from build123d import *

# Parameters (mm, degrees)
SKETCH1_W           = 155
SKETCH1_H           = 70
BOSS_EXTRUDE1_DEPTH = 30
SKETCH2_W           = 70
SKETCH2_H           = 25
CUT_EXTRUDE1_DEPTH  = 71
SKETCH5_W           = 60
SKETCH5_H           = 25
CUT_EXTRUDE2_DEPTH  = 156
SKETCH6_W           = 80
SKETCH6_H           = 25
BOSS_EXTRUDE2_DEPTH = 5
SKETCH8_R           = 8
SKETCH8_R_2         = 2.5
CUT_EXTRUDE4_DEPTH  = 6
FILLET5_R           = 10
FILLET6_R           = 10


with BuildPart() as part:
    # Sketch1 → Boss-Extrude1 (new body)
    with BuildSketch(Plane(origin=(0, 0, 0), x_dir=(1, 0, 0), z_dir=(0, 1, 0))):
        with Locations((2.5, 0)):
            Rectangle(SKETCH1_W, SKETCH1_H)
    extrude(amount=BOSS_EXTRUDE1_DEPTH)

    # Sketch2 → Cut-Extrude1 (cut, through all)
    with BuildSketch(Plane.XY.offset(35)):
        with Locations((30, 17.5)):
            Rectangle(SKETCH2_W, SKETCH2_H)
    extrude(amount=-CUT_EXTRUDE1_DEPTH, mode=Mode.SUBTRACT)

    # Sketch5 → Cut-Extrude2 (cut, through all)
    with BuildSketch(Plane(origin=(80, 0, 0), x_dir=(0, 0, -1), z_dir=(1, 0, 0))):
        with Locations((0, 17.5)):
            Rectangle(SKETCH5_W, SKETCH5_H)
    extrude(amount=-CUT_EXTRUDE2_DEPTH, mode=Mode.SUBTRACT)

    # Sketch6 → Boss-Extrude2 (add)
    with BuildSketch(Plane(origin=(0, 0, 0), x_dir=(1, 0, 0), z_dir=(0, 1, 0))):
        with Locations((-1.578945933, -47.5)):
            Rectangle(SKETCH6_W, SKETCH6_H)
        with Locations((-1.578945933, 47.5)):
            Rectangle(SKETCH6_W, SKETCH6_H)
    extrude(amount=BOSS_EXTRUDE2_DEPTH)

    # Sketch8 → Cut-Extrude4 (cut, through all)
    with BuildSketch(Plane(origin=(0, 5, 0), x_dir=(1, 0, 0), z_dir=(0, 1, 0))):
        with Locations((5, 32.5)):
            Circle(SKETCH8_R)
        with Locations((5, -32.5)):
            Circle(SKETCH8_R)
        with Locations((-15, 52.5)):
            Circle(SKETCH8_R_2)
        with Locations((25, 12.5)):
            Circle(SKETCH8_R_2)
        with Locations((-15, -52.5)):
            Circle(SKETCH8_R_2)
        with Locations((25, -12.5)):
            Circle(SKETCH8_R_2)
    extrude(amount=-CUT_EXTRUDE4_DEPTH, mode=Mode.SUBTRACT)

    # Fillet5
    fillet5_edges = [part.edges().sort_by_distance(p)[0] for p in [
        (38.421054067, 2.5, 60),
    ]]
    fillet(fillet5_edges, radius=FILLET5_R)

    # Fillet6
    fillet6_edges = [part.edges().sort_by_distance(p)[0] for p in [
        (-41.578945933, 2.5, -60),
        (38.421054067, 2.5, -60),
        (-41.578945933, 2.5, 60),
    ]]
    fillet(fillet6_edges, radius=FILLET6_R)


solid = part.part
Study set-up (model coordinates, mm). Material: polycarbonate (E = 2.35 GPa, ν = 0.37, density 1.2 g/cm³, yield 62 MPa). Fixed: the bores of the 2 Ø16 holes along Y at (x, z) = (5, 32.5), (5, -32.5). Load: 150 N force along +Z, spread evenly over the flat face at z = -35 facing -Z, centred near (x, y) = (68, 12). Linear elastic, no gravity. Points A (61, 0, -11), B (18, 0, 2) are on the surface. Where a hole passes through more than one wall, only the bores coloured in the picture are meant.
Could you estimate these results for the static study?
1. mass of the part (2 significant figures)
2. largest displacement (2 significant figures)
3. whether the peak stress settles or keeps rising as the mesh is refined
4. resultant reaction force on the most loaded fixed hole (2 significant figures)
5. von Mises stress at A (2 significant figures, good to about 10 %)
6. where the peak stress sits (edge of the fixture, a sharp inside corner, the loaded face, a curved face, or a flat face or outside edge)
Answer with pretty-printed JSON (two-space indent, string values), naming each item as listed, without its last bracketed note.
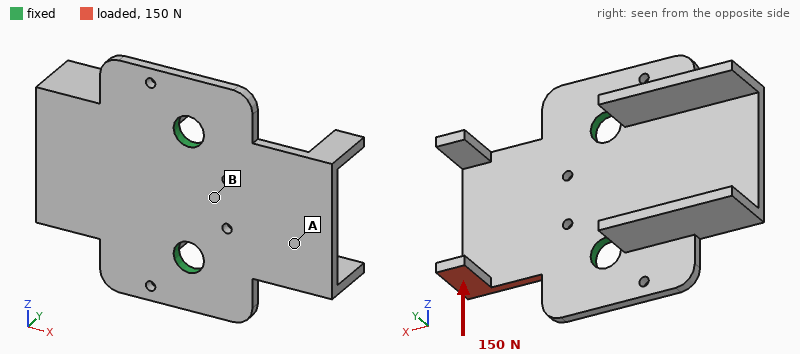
{
  "mass of the part": "110 g",
  "largest displacement": "2.4 mm",
  "whether the peak stress settles or keeps rising as the mesh is refined": "keeps rising",
  "resultant reaction force on the most loaded fixed hole": "150 N",
  "von Mises stress at A": "4.2 MPa",
  "where the peak stress sits": "a sharp inside corner"
}
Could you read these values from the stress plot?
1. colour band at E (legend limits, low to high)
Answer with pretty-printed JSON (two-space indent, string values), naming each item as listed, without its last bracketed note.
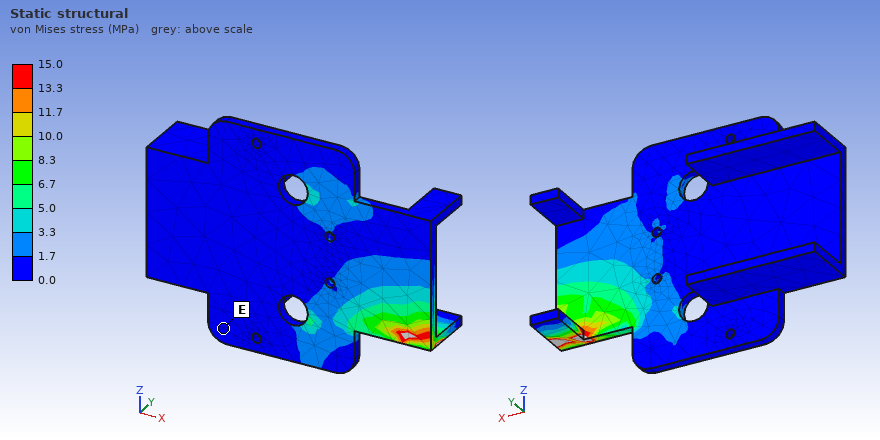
{
  "colour band at E": "0.0 to 1.7 MPa"
}
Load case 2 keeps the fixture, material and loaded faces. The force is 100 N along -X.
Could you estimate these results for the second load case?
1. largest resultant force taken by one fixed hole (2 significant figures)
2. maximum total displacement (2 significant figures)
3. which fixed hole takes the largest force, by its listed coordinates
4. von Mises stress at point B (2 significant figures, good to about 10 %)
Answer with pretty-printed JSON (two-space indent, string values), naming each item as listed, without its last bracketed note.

{
  "largest resultant force taken by one fixed hole": "100 N",
  "maximum total displacement": "2.1 mm",
  "which fixed hole takes the largest force, by its listed coordinates": "(5, -32.5)",
  "von Mises stress at point B": "1.9 MPa"
}
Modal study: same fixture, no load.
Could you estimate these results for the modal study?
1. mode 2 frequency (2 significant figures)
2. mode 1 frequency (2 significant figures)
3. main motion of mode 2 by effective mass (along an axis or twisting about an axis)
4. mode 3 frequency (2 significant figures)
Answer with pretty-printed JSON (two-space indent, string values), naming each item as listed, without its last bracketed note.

{
  "mode 2 frequency": "250 Hz",
  "mode 1 frequency": "210 Hz",
  "main motion of mode 2 by effective mass": "along Y",
  "mode 3 frequency": "400 Hz"
}
